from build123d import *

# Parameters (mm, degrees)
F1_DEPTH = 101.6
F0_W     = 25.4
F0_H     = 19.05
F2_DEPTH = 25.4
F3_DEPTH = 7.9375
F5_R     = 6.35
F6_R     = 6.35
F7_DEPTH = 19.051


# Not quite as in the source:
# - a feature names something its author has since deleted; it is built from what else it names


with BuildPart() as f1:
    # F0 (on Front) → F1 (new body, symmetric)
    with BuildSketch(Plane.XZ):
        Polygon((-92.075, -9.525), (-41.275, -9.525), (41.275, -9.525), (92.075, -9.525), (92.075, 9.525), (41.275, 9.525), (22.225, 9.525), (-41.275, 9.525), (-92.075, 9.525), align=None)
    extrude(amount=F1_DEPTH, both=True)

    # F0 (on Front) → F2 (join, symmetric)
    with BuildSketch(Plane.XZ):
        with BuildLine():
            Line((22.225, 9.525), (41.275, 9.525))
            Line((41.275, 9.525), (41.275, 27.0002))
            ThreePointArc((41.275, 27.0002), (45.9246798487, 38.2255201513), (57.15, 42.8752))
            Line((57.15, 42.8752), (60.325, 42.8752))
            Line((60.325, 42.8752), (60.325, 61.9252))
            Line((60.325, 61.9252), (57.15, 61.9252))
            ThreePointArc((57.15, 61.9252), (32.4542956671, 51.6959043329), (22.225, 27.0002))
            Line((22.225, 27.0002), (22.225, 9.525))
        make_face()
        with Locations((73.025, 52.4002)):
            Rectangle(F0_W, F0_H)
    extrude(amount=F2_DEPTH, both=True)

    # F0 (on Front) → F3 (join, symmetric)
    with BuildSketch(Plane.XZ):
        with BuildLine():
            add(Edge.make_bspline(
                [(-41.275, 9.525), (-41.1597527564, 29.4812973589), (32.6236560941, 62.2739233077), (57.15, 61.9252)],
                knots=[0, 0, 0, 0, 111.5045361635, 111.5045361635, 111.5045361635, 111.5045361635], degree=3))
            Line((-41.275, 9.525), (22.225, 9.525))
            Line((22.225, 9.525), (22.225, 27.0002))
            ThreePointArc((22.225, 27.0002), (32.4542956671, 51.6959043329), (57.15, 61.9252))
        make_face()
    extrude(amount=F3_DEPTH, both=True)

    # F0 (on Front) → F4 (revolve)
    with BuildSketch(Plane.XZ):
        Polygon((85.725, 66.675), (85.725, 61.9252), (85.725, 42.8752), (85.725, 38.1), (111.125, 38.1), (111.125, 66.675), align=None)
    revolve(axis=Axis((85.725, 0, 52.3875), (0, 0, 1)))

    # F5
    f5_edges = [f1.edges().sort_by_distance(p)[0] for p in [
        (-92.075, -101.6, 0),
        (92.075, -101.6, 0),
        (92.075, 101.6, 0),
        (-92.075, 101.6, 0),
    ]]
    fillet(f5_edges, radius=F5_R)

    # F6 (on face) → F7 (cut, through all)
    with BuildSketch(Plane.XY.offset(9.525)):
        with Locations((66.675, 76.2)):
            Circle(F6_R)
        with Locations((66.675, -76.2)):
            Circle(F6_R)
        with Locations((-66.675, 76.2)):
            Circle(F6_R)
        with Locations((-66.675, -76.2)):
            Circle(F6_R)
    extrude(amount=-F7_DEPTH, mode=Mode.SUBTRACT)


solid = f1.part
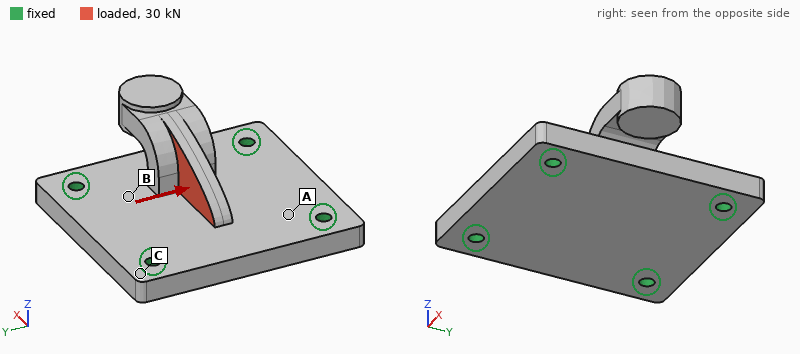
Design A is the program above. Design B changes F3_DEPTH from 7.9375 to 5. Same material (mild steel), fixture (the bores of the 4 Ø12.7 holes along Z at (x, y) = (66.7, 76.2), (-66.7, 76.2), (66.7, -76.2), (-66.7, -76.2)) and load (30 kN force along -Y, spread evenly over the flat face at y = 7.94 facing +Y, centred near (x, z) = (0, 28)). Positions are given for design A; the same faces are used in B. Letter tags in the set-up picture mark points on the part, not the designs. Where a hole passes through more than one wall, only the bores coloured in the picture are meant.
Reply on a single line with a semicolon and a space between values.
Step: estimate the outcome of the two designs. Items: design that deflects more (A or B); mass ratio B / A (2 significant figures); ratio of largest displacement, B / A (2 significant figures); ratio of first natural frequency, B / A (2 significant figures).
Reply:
B; 0.99; 1.7; 0.97
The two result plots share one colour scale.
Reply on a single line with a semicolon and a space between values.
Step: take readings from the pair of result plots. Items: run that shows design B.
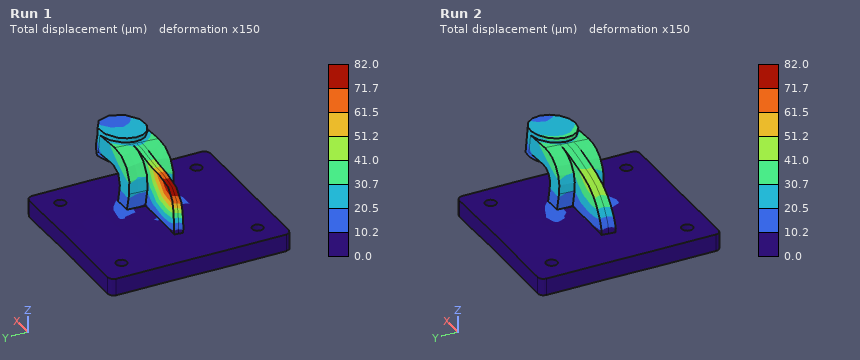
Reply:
Run 1
